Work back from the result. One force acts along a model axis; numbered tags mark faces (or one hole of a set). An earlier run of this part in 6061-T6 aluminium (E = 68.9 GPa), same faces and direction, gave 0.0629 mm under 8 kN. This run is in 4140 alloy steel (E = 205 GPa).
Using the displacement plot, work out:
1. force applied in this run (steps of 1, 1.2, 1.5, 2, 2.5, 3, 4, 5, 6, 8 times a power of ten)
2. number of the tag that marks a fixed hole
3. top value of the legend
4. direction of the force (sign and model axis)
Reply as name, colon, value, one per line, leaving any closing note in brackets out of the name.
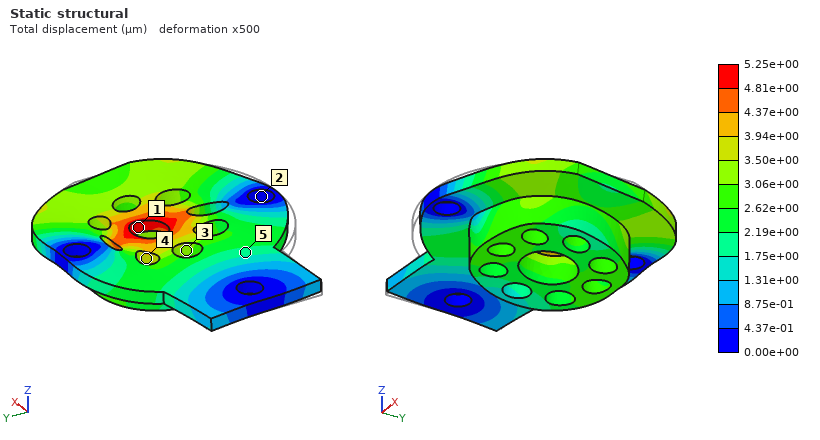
force applied in this run: 2 kN
number of the tag that marks a fixed hole: 2
top value of the legend: 5.25e+00 µm
direction of the force: +Y
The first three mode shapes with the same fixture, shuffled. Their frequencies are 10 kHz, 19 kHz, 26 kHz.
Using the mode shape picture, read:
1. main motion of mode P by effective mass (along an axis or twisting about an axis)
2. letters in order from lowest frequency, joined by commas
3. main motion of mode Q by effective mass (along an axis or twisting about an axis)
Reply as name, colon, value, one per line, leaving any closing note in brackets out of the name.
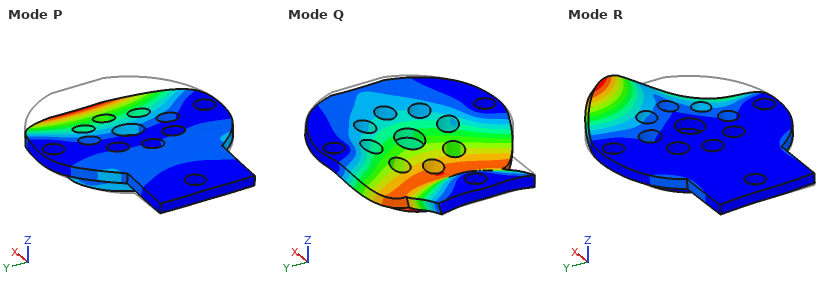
main motion of mode P by effective mass: along Z
letters in order from lowest frequency, joined by commas: P, Q, R
main motion of mode Q by effective mass: along Z
